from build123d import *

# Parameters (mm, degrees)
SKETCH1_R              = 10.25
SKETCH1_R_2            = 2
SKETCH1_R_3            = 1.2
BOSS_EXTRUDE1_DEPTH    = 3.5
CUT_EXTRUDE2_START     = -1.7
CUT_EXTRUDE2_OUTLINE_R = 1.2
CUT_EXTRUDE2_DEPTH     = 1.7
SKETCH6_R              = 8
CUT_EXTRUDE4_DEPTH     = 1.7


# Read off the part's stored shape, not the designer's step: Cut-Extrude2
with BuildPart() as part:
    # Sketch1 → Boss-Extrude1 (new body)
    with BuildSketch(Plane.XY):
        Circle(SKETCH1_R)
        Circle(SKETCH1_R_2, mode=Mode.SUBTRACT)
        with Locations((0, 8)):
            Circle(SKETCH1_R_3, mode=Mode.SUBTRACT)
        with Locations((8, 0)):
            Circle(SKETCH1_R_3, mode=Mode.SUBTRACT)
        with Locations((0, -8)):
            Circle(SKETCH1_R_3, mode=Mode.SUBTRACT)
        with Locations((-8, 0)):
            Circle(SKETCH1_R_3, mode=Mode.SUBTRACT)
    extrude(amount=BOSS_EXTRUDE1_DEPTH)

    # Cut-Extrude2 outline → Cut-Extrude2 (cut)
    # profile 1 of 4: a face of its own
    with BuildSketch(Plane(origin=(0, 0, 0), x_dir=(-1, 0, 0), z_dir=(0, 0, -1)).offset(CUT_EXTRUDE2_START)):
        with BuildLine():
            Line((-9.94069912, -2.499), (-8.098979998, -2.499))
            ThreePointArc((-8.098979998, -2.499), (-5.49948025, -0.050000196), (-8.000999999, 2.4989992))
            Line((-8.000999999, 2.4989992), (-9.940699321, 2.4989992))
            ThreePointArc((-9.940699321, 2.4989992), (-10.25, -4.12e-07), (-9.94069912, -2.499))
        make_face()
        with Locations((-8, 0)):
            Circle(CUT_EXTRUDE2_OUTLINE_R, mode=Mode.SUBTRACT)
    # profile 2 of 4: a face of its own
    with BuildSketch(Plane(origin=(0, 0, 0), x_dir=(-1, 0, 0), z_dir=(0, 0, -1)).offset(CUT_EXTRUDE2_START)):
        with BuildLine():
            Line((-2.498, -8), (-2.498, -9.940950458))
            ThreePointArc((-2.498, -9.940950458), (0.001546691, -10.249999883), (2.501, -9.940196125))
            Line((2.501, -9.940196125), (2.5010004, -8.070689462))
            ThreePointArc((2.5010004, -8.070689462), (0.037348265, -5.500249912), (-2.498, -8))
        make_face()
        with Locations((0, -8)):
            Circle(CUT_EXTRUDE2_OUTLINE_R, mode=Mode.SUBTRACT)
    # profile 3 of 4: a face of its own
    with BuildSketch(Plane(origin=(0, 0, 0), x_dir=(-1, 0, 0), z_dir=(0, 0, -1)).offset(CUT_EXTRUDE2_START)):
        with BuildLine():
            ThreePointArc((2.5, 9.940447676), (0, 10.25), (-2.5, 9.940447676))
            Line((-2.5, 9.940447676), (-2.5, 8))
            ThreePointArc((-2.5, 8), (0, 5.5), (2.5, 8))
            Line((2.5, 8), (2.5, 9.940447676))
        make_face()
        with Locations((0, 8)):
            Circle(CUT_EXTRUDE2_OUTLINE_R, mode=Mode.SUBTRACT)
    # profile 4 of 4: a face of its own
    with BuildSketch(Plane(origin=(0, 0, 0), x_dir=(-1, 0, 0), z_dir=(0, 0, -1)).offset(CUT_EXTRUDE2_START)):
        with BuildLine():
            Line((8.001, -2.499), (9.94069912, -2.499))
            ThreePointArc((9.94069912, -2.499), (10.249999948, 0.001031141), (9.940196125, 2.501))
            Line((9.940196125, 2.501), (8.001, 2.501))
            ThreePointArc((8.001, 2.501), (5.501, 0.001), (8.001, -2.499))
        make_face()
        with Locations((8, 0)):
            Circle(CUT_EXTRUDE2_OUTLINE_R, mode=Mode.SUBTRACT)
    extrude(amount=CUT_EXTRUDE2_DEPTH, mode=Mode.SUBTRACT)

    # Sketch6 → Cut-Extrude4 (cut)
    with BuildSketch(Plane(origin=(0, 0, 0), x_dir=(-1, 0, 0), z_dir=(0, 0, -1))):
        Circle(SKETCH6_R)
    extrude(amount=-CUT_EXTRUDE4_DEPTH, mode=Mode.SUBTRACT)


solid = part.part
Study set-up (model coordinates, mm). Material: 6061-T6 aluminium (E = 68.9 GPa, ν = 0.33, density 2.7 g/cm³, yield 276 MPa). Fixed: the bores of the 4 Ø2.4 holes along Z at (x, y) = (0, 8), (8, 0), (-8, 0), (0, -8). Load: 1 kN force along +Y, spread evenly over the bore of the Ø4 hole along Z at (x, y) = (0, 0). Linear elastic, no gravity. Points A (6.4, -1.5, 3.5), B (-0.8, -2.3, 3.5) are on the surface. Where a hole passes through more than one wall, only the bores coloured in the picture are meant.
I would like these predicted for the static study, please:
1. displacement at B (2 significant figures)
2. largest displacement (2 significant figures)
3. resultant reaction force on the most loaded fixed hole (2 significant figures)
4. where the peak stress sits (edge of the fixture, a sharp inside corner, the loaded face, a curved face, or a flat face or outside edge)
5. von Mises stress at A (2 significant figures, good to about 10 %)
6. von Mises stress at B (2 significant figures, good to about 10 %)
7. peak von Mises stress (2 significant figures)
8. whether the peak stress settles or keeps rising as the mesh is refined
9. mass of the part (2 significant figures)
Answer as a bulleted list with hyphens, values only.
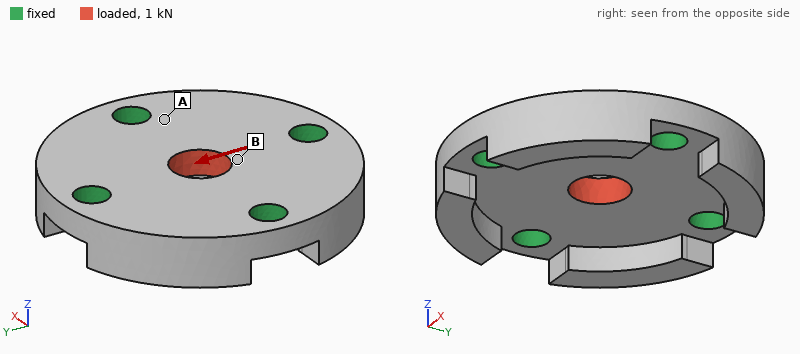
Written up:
- 3.0 µm
- 3.7 µm
- 330 N
- the loaded face
- 14 MPa
- 48 MPa
- 77 MPa
- settles
- 1.8 g
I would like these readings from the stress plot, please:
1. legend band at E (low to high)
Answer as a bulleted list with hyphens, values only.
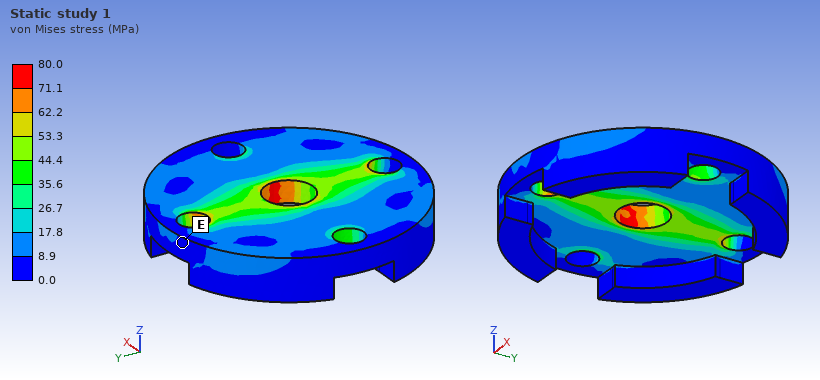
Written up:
- 0.0 to 8.9 MPa
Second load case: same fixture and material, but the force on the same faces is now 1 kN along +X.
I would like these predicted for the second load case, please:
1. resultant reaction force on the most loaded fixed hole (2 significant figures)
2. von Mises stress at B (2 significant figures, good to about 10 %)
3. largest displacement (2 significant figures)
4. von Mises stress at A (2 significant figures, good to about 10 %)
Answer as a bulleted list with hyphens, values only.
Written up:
- 330 N
- 44 MPa
- 3.7 µm
- 29 MPa
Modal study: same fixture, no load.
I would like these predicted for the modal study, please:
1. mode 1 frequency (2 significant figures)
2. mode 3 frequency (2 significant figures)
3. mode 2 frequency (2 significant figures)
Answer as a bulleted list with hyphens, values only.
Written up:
- 49 kHz
- 51 kHz
- 50 kHz
